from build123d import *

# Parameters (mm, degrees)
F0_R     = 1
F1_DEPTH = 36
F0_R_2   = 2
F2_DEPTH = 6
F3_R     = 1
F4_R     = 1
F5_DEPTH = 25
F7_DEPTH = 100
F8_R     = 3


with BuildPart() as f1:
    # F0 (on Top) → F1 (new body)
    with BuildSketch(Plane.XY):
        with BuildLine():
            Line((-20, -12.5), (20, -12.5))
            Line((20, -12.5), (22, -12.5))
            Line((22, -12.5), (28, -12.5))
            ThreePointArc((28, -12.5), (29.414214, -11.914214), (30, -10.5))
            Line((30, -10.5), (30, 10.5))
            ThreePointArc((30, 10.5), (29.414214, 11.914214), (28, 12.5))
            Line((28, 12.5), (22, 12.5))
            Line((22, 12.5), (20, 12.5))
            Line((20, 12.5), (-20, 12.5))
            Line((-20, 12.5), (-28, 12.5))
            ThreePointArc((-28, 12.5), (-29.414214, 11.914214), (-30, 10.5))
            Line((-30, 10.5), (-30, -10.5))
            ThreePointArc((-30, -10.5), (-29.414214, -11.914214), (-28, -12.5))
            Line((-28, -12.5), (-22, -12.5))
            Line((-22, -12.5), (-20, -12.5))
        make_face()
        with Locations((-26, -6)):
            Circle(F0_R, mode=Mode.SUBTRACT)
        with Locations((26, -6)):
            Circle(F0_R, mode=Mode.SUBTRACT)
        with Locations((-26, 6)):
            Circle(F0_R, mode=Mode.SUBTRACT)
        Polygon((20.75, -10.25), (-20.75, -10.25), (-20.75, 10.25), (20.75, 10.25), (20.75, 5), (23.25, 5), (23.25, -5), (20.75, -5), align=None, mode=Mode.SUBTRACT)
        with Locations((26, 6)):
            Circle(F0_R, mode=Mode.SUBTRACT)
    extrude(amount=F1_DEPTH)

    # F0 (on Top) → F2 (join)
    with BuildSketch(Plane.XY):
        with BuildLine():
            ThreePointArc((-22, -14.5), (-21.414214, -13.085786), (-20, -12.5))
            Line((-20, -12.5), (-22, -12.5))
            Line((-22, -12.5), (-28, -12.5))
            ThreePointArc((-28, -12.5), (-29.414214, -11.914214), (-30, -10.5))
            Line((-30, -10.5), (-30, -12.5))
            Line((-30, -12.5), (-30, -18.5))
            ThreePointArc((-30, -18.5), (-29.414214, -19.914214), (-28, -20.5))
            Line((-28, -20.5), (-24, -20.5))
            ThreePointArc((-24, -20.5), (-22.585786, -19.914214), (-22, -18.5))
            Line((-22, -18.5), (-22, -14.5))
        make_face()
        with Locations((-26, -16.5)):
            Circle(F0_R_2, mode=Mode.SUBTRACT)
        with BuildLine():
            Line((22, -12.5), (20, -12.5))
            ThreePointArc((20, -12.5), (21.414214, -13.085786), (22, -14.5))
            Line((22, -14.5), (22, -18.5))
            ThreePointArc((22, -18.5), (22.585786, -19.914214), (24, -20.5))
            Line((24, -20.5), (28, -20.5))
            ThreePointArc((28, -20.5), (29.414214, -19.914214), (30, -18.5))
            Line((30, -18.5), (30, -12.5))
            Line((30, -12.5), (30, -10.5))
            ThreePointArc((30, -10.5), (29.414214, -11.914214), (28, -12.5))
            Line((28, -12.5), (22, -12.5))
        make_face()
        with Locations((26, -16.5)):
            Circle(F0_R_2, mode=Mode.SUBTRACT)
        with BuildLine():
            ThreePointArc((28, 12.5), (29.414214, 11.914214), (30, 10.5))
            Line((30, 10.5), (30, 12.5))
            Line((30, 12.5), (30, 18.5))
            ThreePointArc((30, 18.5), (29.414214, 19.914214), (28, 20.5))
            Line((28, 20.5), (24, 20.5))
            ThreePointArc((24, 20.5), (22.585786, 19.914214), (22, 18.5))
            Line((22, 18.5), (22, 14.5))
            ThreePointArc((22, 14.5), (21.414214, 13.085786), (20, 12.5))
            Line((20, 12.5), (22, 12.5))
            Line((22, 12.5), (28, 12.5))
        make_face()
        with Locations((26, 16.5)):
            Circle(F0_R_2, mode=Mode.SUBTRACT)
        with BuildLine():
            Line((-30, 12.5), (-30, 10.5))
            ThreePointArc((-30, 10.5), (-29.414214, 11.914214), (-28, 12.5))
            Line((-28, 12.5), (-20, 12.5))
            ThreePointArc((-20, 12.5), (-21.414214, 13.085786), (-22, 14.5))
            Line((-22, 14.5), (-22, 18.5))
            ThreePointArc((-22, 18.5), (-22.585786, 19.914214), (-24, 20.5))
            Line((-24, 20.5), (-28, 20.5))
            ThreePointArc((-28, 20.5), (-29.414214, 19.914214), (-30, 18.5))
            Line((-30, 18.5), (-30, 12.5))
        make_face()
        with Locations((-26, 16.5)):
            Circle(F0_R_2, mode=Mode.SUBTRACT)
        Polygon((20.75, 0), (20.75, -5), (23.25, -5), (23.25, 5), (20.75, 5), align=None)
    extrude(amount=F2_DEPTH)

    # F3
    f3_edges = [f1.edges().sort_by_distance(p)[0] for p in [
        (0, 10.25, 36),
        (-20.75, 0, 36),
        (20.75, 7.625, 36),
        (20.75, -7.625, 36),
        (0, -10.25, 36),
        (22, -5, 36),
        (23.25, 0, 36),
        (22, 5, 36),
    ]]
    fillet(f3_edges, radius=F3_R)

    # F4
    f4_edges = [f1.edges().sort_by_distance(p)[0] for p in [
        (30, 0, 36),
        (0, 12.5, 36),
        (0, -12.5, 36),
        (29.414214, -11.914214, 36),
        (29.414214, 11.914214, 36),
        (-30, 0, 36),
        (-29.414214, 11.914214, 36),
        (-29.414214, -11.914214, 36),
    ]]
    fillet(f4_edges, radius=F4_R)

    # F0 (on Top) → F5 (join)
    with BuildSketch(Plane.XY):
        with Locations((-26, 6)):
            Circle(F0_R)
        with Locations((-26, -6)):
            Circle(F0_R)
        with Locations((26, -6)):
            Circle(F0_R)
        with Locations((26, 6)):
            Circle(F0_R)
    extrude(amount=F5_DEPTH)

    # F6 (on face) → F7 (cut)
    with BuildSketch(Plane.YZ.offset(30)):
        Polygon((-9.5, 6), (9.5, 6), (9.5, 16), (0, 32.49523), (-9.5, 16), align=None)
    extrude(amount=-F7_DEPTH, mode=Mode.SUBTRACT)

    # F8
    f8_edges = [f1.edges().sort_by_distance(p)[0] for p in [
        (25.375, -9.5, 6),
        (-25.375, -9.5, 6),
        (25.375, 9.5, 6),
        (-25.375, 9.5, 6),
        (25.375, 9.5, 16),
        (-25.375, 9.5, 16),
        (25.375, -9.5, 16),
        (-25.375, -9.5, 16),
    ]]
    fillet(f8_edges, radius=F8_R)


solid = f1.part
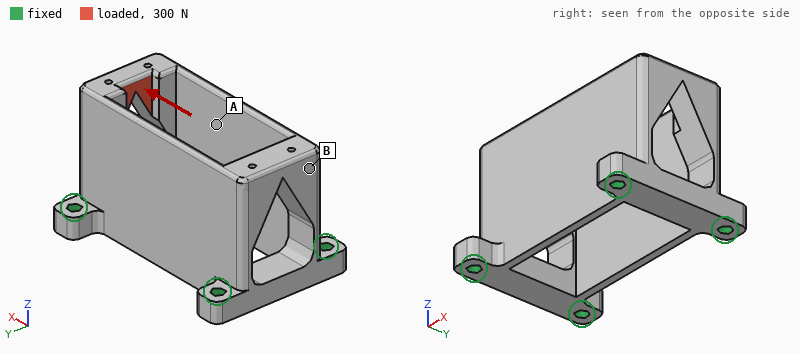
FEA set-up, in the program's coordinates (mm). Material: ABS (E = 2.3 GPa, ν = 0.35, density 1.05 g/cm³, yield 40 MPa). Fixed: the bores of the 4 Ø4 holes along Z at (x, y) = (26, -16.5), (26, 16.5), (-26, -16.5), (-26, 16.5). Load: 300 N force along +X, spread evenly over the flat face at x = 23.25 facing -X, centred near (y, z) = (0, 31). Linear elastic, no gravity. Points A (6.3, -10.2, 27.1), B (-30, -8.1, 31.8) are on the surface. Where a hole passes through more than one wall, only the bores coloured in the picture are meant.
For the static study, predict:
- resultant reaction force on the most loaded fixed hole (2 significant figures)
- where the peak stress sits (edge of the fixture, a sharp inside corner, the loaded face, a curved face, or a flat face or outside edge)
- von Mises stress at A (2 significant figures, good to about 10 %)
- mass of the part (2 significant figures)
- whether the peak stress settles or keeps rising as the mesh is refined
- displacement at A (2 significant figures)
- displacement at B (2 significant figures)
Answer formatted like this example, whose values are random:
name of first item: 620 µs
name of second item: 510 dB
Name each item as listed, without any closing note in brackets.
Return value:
resultant reaction force on the most loaded fixed hole: 120 N
where the peak stress sits: a sharp inside corner
von Mises stress at A: 5.0 MPa
mass of the part: 19 g
whether the peak stress settles or keeps rising as the mesh is refined: keeps rising
displacement at A: 0.21 mm
displacement at B: 0.058 mm
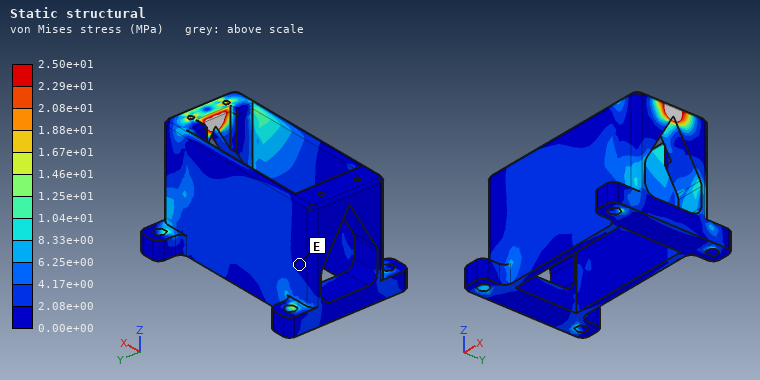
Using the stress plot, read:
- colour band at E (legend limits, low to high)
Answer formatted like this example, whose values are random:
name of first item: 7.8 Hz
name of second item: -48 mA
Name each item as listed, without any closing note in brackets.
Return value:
colour band at E: 0.00e+00 to 2.08e+00 MPa
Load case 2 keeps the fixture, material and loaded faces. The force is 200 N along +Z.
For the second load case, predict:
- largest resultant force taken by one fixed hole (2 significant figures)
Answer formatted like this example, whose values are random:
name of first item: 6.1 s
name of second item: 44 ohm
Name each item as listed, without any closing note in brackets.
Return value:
largest resultant force taken by one fixed hole: 99 N
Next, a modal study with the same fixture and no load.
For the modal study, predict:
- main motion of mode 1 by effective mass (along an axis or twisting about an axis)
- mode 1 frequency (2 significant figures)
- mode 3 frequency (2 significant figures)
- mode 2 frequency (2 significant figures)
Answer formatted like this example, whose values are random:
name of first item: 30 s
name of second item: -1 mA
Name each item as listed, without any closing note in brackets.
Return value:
main motion of mode 1 by effective mass: along Y
mode 1 frequency: 1300 Hz
mode 3 frequency: 1600 Hz
mode 2 frequency: 1600 Hz
